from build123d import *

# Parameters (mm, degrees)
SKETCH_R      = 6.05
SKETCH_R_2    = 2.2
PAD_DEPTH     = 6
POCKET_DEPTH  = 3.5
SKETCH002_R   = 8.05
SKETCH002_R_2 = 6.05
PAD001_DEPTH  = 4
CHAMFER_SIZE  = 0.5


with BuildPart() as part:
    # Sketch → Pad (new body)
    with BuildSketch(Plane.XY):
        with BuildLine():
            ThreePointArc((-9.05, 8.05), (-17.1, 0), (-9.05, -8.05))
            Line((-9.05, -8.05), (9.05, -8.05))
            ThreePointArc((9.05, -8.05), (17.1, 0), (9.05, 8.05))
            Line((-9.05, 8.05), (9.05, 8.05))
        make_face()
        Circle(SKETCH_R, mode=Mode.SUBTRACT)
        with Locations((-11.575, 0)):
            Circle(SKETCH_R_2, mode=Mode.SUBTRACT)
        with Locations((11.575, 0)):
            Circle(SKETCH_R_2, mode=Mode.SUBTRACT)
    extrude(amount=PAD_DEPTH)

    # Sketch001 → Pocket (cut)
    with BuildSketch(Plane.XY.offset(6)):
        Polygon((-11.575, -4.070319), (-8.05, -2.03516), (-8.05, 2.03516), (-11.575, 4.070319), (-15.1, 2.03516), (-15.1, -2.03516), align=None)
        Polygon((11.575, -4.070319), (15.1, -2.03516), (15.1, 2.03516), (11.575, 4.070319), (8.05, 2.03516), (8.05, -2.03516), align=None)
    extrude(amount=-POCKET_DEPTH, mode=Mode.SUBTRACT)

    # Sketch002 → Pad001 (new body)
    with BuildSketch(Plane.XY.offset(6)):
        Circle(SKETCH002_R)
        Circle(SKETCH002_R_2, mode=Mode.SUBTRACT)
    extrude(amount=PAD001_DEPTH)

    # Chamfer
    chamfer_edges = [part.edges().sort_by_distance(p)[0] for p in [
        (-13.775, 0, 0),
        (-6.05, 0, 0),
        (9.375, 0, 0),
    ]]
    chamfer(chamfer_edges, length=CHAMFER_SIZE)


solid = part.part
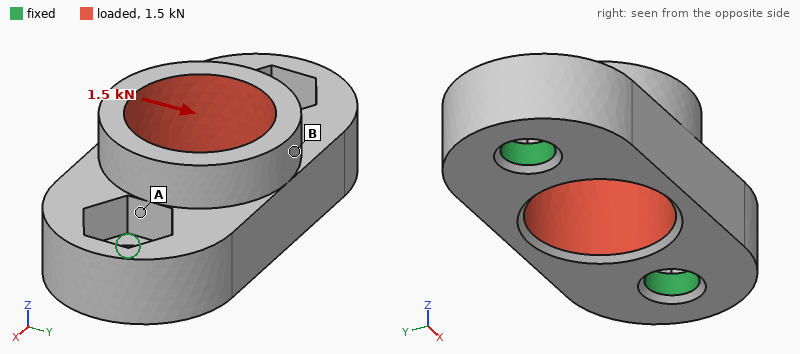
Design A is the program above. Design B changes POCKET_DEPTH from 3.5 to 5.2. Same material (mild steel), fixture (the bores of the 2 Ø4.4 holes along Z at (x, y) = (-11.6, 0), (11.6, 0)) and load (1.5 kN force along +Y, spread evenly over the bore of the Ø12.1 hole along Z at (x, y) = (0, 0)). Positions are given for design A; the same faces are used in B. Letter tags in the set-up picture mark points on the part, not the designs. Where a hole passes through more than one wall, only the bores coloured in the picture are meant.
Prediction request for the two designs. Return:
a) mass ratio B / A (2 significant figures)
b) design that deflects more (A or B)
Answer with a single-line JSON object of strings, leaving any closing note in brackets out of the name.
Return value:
{"mass ratio B / A": "0.96", "design that deflects more": "B"}
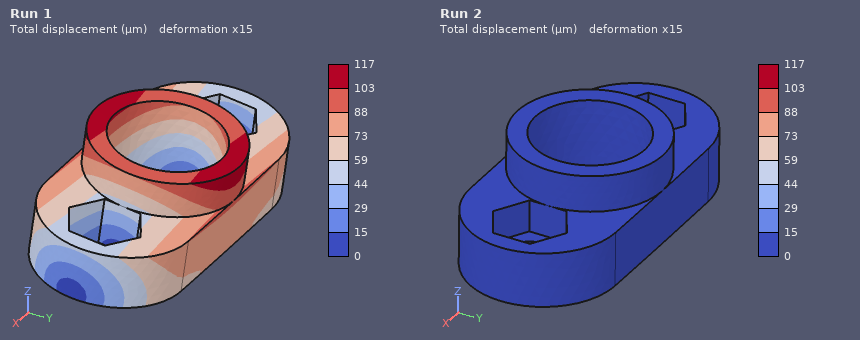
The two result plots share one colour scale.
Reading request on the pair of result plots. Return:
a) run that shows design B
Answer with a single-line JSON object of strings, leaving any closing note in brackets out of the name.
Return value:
{"run that shows design B": "Run 1"}
